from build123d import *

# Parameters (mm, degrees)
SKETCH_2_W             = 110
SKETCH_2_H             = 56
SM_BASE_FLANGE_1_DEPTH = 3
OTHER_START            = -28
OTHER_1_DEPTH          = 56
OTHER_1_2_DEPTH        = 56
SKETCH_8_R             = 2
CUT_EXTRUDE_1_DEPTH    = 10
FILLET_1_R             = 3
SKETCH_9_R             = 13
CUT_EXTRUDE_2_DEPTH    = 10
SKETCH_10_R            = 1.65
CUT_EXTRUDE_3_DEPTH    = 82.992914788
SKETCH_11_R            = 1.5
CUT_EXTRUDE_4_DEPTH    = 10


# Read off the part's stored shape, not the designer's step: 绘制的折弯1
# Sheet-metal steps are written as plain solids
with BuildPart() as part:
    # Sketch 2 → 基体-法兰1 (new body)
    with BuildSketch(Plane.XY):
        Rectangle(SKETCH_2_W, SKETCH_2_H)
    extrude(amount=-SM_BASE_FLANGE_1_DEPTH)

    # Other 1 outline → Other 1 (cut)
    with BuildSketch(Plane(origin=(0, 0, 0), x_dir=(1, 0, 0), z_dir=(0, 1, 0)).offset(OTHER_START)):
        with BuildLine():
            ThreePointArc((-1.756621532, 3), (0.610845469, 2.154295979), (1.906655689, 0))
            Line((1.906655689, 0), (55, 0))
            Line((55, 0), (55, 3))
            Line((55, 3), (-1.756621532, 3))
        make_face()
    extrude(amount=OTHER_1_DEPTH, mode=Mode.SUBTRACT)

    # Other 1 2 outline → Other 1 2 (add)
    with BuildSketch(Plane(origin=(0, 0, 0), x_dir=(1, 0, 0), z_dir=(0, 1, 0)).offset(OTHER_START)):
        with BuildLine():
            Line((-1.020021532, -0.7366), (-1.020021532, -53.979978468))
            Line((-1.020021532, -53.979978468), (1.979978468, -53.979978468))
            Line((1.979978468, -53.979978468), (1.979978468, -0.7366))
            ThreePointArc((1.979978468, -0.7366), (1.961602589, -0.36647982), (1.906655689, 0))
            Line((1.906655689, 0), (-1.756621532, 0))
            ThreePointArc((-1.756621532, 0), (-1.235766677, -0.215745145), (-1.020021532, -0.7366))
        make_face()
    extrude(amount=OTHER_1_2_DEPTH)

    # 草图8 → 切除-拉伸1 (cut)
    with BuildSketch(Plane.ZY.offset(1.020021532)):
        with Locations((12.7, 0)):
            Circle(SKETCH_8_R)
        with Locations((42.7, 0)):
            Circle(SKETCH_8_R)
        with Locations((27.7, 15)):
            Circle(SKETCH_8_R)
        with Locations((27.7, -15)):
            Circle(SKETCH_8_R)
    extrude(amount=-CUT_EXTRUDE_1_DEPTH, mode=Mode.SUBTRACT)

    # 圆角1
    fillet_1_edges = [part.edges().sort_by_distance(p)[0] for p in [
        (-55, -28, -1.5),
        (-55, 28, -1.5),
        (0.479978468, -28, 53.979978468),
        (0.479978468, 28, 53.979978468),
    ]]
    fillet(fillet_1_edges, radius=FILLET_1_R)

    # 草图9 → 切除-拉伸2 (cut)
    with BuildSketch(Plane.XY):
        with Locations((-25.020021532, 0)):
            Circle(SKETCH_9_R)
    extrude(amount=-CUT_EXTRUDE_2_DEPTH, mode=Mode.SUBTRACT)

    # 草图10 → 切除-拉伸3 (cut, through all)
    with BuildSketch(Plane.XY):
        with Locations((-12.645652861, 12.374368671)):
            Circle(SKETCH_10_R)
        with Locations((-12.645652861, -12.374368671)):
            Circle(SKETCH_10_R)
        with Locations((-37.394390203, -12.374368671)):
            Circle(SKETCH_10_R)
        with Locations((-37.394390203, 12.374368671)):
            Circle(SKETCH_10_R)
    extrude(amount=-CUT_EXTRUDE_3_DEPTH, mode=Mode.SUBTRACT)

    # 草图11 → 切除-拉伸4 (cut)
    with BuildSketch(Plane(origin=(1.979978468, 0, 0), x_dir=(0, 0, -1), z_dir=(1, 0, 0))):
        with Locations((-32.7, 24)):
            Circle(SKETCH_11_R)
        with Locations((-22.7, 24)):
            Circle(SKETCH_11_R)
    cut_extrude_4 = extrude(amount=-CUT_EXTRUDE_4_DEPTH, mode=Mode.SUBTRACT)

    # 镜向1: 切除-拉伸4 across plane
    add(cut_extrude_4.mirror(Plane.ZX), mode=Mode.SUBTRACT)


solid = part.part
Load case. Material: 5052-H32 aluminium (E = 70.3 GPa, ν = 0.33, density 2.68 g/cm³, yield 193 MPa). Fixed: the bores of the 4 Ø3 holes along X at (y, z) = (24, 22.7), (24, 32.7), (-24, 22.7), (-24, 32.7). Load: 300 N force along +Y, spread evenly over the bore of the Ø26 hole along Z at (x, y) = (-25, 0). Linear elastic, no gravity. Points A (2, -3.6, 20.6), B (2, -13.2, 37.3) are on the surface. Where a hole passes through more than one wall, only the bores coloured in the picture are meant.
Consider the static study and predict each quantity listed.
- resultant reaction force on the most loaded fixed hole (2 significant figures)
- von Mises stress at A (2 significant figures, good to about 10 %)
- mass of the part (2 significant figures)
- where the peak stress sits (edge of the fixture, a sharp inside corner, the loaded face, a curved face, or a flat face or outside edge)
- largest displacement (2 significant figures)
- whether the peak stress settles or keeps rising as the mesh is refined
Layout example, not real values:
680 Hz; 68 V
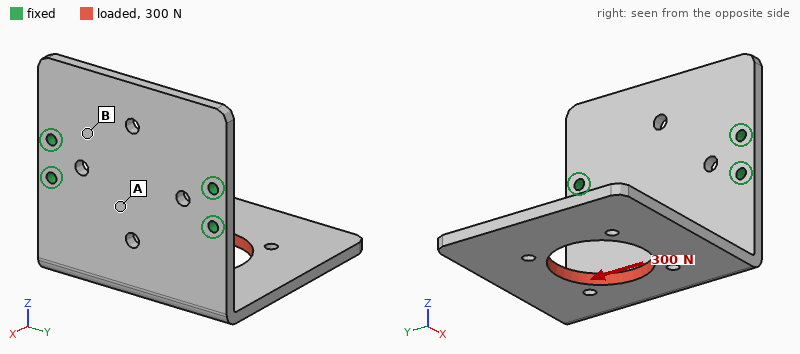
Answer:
270 N; 13 MPa; 44 g; edge of the fixture; 0.33 mm; keeps rising
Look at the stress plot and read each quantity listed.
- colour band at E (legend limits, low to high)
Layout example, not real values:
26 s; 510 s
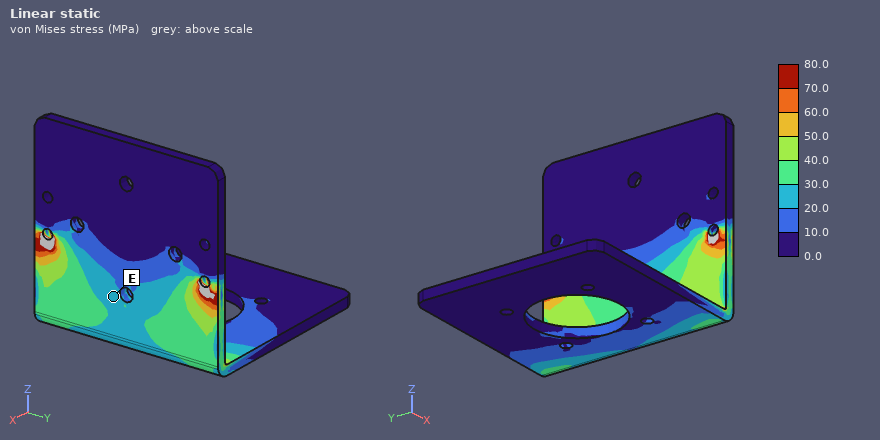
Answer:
20.0 to 30.0 MPa
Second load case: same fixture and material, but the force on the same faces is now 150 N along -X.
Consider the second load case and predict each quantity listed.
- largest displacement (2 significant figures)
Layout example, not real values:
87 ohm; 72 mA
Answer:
0.35 mm
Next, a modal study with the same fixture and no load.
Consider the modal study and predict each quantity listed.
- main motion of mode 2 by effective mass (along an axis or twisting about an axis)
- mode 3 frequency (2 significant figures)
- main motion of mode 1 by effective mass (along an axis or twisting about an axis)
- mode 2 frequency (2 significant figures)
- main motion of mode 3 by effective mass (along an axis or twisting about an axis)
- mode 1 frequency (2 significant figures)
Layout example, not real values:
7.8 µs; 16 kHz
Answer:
along Y; 1600 Hz; along Z; 1100 Hz; along X; 470 Hz
